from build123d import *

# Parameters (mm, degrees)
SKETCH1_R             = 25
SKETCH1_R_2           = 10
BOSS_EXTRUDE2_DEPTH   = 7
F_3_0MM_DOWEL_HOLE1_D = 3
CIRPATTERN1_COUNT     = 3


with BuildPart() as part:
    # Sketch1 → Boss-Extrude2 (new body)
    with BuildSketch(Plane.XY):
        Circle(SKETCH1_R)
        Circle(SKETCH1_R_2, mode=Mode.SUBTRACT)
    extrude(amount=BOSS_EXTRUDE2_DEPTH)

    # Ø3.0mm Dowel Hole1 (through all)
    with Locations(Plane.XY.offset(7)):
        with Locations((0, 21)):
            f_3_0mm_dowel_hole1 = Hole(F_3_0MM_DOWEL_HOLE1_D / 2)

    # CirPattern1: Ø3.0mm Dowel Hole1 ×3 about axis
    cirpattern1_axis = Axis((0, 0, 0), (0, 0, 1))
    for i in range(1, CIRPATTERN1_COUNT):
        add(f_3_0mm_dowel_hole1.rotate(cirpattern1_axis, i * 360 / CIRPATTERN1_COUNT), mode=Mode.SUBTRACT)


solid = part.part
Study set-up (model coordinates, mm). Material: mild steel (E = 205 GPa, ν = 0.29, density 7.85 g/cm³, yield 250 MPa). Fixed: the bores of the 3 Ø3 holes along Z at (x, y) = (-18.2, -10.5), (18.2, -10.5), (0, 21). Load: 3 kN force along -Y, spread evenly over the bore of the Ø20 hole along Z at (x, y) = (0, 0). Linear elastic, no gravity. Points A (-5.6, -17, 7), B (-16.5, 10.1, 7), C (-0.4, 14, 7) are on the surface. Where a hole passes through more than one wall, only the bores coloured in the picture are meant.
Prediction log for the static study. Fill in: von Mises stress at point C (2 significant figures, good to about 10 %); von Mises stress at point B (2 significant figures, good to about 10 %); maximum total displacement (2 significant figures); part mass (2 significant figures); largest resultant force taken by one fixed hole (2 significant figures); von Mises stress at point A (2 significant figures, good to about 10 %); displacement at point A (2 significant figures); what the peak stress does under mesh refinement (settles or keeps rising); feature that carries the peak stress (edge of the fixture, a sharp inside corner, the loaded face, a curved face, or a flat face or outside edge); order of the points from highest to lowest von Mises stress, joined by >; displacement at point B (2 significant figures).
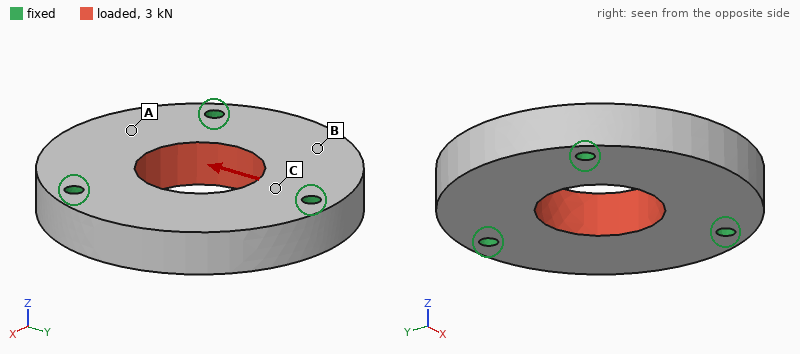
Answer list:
12 MPa
4.0 MPa
1.6 µm
89 g
1.1 kN
7.4 MPa
1.3 µm
keeps rising
edge of the fixture
C > A > B
0.76 µm
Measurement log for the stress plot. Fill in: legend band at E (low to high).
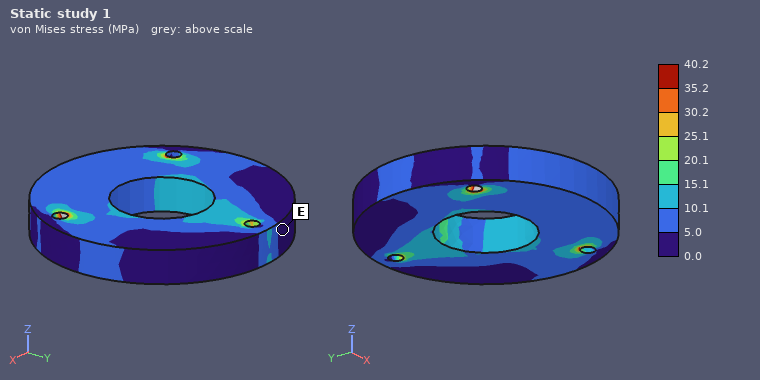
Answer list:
0.0 to 5.0 MPa
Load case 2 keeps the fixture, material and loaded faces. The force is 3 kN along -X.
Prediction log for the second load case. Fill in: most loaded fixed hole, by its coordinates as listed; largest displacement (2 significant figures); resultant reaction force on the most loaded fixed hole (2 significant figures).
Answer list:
(0, 21)
1.5 µm
1.1 kN
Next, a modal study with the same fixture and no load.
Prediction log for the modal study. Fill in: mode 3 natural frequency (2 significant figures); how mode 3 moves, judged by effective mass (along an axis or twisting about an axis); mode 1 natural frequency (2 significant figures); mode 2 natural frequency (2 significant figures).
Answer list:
18 kHz
along Z
15 kHz
15 kHz
